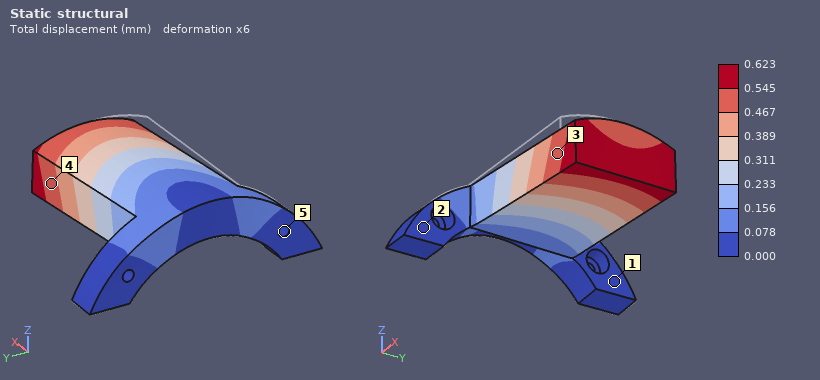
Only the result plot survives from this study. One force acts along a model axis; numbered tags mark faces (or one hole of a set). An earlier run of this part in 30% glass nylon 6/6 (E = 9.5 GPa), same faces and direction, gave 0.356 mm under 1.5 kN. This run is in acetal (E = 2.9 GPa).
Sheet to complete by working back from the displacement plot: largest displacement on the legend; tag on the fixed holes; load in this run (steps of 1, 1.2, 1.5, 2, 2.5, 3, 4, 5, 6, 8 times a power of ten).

0.623 mm
5
800 N
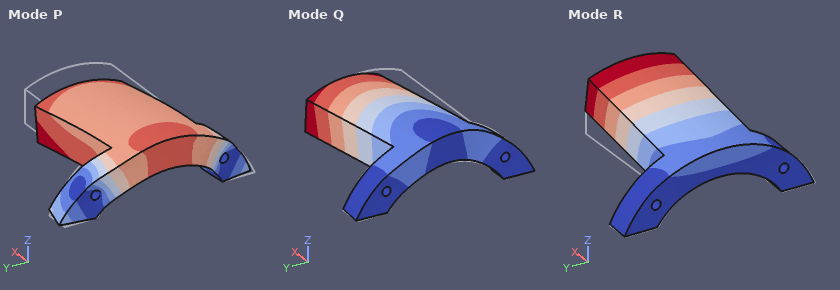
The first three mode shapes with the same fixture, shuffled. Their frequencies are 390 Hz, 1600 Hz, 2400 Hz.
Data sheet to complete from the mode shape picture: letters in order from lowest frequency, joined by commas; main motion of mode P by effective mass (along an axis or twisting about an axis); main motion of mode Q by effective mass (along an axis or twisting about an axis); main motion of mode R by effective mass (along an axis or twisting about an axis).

R, Q, P
along X
along Y
along Z
